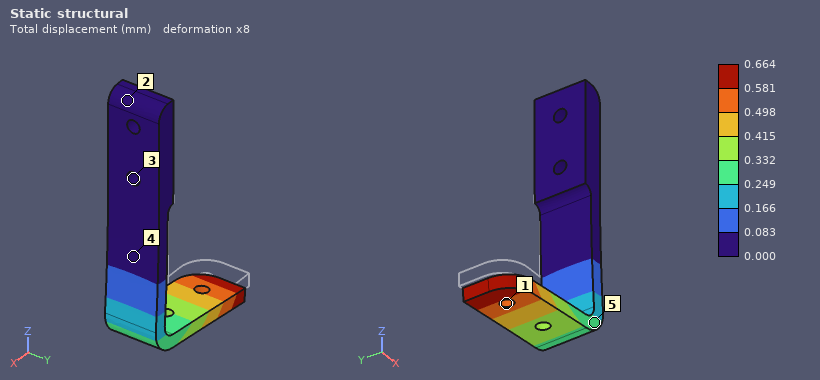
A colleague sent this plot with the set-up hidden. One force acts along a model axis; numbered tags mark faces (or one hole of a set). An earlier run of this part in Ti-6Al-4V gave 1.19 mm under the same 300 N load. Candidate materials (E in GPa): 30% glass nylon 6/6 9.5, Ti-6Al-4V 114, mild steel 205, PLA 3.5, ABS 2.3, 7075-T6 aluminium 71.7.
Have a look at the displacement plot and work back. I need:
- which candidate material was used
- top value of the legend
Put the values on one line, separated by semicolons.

mild steel; 0.664 mm
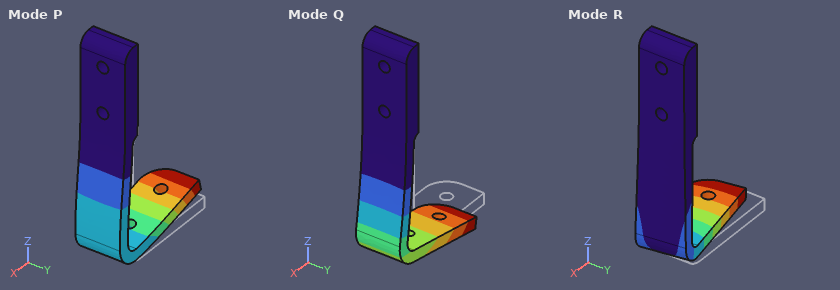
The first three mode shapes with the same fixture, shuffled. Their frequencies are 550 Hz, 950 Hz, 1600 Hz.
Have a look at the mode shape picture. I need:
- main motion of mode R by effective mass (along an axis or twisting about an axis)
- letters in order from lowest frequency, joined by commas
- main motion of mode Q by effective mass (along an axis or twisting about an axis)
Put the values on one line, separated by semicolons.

along Y; Q, R, P; along X
